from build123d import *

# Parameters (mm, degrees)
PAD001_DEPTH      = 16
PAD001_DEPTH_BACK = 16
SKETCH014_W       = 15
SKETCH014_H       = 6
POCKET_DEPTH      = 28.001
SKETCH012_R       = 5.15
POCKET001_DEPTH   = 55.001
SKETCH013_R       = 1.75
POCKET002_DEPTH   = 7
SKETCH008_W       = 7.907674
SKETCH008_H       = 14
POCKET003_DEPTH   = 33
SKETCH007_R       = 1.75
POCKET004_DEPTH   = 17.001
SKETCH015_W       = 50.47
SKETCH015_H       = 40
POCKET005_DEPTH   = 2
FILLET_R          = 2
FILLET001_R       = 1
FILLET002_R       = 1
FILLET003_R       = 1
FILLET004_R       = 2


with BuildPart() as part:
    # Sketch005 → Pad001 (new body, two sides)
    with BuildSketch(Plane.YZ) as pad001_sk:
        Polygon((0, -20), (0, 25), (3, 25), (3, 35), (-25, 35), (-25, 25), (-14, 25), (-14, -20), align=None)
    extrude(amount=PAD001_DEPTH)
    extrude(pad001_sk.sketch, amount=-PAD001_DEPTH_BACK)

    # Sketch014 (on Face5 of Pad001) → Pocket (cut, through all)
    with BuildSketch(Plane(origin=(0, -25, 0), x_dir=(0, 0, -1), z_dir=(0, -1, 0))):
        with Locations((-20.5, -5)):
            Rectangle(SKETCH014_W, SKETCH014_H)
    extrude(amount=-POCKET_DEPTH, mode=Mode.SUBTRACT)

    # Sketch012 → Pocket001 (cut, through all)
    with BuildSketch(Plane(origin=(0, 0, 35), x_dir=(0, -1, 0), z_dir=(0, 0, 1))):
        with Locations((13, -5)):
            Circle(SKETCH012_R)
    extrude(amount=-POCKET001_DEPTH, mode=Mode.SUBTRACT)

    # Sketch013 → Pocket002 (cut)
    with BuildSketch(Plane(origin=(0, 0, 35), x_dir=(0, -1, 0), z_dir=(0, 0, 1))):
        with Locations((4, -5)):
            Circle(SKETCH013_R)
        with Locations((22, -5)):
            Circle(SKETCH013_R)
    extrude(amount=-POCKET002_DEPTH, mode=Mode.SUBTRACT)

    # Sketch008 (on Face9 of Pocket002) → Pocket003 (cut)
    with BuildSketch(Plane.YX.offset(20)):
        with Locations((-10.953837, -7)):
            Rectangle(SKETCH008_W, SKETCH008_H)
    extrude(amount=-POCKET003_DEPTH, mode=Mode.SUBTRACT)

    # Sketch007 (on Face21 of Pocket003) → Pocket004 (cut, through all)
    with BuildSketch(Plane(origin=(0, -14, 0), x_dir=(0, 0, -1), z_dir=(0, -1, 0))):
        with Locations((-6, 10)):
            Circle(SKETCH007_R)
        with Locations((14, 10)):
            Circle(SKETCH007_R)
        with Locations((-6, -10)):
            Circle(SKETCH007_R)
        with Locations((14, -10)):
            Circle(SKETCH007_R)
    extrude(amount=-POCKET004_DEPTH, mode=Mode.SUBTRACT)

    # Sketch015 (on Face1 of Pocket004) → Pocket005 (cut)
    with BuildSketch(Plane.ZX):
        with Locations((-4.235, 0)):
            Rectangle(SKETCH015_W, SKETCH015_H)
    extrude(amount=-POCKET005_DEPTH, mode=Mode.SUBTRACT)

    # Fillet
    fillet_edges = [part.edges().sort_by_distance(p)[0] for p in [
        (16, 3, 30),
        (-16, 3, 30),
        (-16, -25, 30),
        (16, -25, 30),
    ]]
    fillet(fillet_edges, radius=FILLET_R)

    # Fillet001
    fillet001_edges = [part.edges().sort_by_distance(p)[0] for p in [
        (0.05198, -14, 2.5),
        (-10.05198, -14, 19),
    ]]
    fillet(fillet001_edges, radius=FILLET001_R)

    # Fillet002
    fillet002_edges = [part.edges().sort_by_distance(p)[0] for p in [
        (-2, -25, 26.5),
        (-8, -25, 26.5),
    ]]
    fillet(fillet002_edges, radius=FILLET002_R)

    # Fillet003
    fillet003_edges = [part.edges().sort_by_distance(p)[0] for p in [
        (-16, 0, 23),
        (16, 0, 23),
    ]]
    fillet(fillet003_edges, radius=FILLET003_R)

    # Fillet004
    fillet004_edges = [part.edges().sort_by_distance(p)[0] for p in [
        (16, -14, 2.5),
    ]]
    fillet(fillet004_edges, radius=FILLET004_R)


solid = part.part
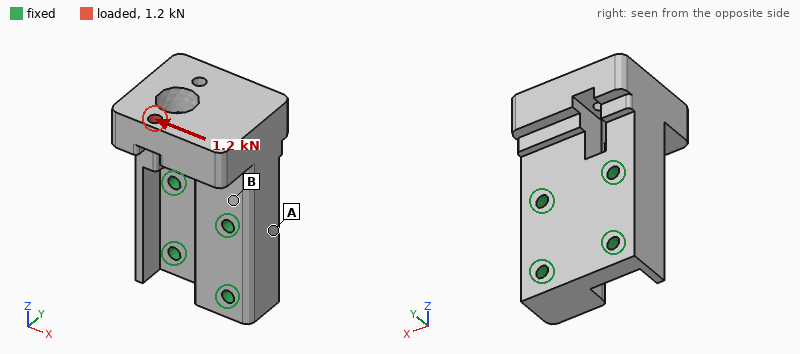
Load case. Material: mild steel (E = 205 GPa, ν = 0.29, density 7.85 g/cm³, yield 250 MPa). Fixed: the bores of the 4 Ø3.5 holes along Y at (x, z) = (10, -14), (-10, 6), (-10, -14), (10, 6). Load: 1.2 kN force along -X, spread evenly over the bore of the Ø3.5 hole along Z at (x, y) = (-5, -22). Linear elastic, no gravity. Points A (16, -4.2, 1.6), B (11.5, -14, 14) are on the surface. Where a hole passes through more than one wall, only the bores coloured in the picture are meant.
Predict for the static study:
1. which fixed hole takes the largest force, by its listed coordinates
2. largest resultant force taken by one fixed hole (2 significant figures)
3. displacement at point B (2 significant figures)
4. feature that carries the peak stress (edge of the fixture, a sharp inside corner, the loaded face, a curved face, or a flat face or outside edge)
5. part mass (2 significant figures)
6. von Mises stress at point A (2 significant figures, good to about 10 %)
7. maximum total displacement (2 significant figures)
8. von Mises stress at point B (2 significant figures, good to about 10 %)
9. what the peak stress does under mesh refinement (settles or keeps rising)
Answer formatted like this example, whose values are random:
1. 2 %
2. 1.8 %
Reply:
1. (10, 6)
2. 1.7 kN
3. 2.6 µm
4. edge of the fixture
5. 160 g
6. 14 MPa
7. 17 µm
8. 32 MPa
9. keeps rising
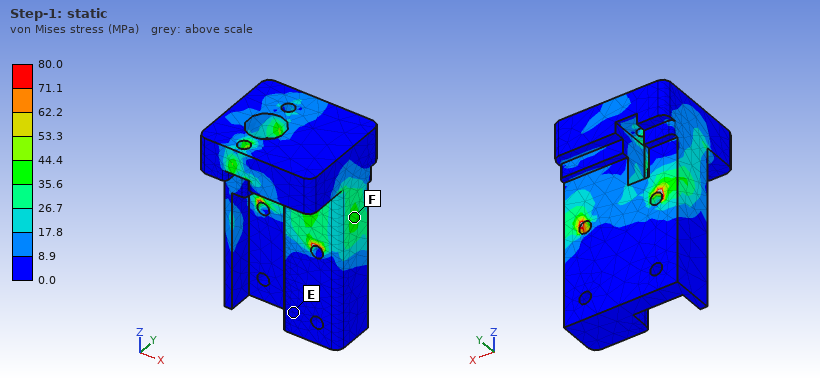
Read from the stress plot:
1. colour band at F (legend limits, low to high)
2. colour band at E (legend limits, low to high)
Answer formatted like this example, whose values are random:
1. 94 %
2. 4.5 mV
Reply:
1. 35.6 to 44.4 MPa
2. 0.0 to 8.9 MPa
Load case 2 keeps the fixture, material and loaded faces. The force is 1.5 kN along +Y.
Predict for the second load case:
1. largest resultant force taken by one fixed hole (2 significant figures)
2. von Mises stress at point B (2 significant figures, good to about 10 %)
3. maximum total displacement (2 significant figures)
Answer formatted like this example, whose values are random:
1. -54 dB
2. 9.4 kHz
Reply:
1. 1.1 kN
2. 57 MPa
3. 37 µm
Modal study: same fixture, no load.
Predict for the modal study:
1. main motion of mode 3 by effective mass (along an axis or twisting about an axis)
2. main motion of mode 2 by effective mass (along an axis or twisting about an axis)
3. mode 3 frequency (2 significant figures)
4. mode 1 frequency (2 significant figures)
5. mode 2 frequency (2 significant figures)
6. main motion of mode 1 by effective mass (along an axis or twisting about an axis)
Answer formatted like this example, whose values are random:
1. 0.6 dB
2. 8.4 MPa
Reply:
1. along X
2. along X
3. 11 kHz
4. 5300 Hz
5. 8200 Hz
6. along Y
